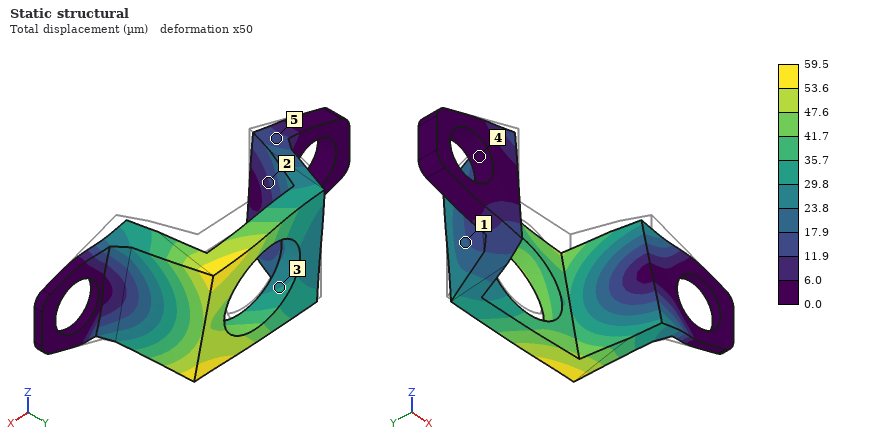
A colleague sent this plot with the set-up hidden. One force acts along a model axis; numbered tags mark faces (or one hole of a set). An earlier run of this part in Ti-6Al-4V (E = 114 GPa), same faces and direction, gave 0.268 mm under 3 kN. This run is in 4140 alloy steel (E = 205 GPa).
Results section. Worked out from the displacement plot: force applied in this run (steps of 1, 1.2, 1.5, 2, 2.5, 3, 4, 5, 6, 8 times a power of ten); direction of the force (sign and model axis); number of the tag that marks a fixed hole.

1.2 kN
-Z
4
